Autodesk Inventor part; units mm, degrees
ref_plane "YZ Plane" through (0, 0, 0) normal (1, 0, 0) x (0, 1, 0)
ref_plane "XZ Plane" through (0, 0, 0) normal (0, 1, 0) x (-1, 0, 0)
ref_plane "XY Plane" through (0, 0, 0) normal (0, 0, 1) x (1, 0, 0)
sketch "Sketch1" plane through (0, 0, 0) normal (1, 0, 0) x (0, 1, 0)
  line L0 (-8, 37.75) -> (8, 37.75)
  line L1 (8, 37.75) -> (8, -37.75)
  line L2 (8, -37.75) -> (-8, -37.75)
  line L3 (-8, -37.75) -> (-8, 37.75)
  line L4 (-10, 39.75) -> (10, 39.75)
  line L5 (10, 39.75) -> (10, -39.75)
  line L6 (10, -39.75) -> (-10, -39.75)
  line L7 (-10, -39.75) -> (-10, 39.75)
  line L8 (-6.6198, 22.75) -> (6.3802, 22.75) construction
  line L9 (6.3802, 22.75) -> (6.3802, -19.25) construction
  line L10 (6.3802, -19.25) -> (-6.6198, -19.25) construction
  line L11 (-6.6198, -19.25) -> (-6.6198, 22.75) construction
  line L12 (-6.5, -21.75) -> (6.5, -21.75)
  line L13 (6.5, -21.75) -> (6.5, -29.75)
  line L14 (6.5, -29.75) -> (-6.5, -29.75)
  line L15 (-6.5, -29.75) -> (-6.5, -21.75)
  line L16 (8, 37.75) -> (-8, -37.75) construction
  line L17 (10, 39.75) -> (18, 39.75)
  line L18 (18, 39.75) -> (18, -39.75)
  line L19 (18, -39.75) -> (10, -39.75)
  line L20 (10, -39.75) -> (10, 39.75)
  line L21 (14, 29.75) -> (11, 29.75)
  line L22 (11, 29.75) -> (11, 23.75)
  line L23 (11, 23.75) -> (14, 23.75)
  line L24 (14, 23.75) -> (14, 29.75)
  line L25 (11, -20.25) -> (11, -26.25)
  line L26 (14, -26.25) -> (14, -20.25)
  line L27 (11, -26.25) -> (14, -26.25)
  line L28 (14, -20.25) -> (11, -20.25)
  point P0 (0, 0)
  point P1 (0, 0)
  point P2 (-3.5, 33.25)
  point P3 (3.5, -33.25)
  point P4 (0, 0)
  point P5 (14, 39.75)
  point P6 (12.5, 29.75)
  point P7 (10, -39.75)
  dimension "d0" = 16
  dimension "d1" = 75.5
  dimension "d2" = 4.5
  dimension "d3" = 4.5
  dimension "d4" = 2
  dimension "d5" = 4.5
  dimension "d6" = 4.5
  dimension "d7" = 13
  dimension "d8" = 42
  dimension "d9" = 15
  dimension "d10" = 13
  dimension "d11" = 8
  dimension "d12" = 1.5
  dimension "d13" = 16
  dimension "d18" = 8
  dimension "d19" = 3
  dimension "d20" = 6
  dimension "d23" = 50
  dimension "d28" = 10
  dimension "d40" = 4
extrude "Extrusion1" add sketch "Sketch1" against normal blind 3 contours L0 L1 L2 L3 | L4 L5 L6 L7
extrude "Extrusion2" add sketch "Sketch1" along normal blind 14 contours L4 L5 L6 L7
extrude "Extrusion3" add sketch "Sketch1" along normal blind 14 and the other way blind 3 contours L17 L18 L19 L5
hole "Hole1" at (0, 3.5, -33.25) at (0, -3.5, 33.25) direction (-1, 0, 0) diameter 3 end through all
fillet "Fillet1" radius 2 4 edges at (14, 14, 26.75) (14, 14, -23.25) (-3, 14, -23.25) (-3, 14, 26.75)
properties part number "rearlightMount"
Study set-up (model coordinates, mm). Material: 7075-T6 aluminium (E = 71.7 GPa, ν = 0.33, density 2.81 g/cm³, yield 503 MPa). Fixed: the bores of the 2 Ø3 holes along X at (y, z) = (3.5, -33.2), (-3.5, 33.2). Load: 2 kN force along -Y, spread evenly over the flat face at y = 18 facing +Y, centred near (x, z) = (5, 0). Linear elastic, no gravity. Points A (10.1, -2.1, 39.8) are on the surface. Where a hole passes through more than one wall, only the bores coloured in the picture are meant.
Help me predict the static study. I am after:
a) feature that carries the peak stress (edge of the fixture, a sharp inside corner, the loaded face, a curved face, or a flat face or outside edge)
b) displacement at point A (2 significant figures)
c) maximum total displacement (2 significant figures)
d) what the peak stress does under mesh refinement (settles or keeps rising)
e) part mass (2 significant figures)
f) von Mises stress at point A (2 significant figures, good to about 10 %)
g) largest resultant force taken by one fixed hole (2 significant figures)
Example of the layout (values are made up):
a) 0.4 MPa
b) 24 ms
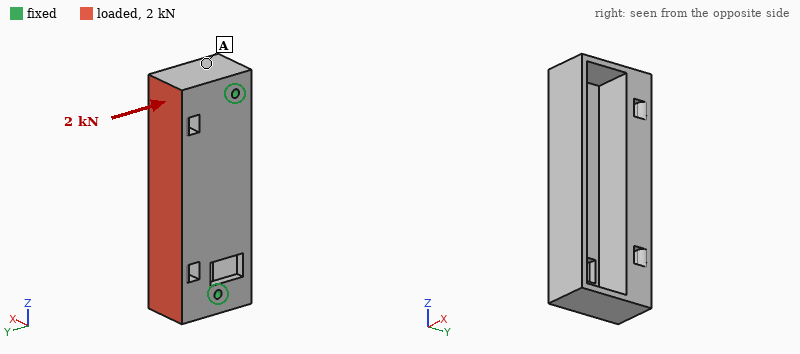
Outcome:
a) edge of the fixture
b) 0.069 mm
c) 0.18 mm
d) keeps rising
e) 56 g
f) 28 MPa
g) 1.1 kN
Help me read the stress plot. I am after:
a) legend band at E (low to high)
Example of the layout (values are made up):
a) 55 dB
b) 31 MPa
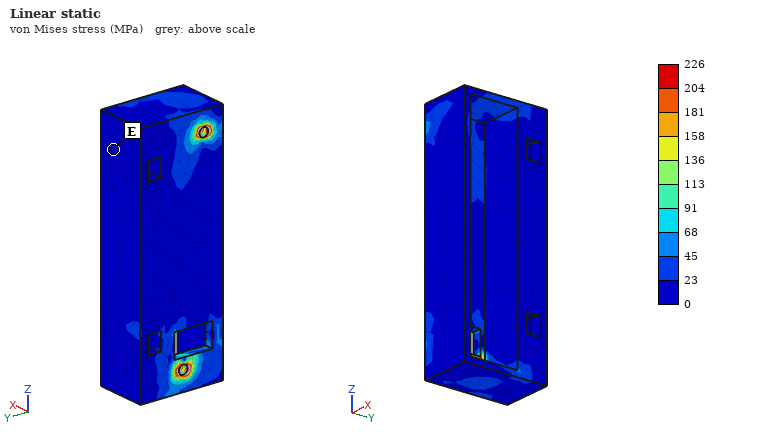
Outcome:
a) 0 to 23 MPa
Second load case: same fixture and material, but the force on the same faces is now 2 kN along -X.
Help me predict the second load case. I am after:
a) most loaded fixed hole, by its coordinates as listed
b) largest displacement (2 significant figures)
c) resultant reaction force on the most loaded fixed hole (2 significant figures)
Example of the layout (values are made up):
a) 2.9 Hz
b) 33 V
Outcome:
a) (3.5, -33.2)
b) 0.43 mm
c) 1.1 kN
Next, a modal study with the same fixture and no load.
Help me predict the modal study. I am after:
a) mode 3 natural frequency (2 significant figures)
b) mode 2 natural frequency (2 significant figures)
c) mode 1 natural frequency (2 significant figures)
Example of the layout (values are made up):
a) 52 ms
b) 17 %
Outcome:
a) 6700 Hz
b) 5400 Hz
c) 2300 Hz
